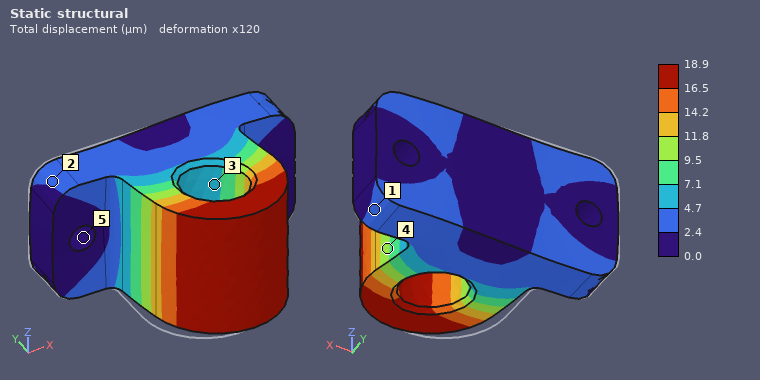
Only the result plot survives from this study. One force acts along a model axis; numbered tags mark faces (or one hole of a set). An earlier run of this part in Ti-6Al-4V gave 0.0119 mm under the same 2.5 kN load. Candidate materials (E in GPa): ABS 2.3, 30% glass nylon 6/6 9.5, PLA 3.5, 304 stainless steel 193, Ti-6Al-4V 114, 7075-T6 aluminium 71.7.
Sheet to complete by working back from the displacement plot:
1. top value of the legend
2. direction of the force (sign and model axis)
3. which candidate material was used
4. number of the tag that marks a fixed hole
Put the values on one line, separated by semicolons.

18.9 µm; +X; 7075-T6 aluminium; 5
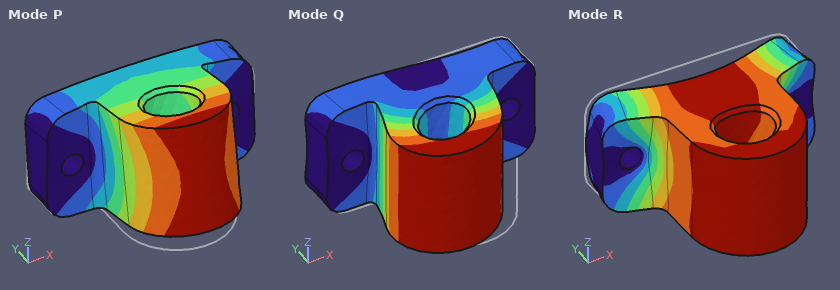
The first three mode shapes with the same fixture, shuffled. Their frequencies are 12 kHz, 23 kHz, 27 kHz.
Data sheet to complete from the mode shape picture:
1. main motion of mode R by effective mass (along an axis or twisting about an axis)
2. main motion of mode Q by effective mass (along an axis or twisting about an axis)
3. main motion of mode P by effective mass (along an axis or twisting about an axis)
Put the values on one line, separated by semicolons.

along Y; along X; along Z
